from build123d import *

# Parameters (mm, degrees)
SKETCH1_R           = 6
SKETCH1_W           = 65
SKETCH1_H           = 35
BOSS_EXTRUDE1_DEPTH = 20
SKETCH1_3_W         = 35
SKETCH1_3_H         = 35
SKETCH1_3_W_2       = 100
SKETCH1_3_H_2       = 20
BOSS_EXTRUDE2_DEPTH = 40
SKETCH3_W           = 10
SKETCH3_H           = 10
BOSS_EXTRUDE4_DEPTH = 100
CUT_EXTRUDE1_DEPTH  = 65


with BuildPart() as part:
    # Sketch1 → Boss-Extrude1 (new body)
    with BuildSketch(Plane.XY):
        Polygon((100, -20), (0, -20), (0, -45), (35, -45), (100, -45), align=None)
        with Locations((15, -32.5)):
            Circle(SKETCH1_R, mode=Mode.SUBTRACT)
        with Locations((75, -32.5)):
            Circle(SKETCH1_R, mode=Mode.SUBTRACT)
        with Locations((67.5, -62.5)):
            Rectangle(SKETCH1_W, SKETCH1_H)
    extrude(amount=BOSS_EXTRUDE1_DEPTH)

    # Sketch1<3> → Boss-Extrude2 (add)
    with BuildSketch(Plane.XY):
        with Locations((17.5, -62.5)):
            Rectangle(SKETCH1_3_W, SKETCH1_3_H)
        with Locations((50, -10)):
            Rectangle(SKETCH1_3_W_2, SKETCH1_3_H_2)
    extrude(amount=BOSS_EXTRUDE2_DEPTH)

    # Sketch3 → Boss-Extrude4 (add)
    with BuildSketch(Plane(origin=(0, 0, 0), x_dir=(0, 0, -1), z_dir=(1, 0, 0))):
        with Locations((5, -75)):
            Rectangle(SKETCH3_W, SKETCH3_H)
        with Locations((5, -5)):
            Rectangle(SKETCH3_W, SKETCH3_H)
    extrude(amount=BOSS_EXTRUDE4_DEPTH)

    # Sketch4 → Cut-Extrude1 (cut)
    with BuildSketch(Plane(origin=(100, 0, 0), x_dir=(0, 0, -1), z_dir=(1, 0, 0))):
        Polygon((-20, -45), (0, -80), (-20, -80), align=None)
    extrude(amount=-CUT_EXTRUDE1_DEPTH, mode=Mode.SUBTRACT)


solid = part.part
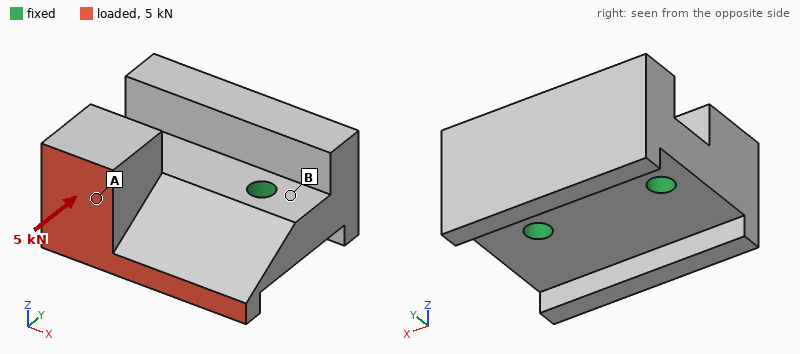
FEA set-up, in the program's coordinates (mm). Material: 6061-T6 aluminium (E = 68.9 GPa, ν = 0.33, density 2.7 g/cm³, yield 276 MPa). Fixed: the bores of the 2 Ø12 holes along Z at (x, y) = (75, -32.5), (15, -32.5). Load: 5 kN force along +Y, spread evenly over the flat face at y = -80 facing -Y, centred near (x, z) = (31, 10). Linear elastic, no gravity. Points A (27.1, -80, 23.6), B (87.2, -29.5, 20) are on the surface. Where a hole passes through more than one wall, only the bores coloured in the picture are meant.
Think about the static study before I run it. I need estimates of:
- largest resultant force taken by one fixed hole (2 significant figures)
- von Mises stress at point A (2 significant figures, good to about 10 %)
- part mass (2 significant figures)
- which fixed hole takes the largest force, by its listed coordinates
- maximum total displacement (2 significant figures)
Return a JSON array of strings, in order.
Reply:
["3.6 kN", "3.6 MPa", "590 g", "(15, -32.5)", "30 µm"]
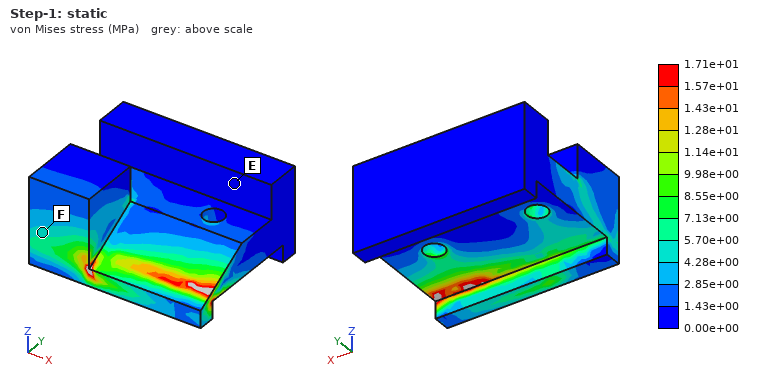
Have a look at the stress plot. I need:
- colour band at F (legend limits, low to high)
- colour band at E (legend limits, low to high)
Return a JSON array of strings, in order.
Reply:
["4.28e+00 to 5.70e+00 MPa", "0.00e+00 to 1.43e+00 MPa"]
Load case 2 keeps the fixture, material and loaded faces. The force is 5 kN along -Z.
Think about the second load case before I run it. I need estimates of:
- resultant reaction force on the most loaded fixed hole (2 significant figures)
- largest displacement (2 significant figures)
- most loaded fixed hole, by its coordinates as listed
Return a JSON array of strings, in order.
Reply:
["3.6 kN", "77 µm", "(15, -32.5)"]
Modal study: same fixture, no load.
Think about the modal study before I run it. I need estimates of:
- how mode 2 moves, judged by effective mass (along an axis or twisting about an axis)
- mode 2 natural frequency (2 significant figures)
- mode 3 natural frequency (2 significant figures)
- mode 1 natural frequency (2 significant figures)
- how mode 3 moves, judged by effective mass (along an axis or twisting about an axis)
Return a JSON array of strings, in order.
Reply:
["along Z", "6400 Hz", "7100 Hz", "4500 Hz", "along Z"]
